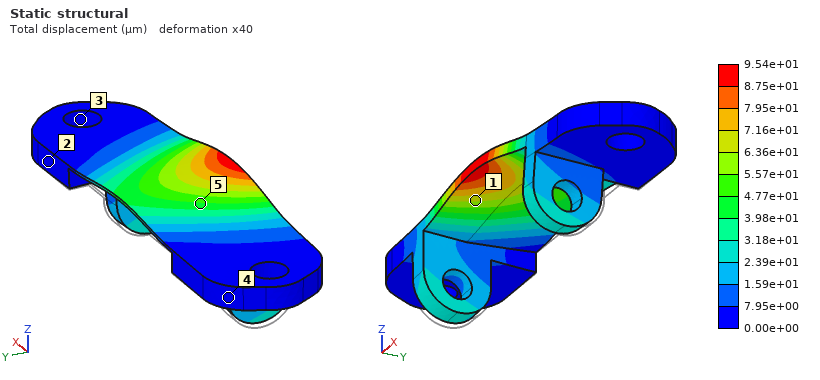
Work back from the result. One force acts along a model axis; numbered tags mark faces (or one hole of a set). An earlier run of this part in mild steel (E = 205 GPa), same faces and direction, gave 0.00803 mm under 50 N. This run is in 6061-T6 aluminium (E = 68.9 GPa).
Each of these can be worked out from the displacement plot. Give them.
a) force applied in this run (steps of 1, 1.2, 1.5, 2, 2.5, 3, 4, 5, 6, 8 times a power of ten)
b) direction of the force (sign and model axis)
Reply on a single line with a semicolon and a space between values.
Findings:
200 N; +Z
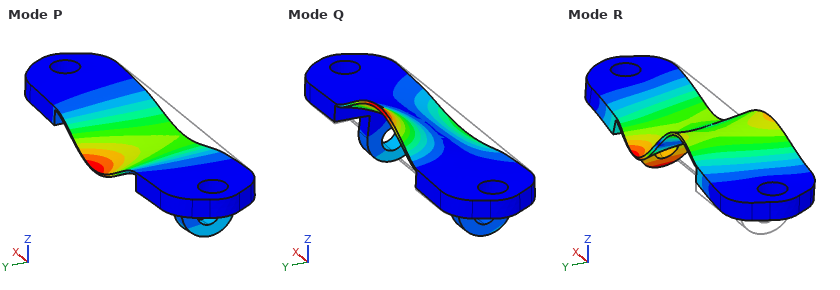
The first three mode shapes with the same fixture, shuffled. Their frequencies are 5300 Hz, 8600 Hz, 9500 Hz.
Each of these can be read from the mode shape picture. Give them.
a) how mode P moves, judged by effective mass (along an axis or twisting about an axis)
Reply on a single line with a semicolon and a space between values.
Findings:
along Z
